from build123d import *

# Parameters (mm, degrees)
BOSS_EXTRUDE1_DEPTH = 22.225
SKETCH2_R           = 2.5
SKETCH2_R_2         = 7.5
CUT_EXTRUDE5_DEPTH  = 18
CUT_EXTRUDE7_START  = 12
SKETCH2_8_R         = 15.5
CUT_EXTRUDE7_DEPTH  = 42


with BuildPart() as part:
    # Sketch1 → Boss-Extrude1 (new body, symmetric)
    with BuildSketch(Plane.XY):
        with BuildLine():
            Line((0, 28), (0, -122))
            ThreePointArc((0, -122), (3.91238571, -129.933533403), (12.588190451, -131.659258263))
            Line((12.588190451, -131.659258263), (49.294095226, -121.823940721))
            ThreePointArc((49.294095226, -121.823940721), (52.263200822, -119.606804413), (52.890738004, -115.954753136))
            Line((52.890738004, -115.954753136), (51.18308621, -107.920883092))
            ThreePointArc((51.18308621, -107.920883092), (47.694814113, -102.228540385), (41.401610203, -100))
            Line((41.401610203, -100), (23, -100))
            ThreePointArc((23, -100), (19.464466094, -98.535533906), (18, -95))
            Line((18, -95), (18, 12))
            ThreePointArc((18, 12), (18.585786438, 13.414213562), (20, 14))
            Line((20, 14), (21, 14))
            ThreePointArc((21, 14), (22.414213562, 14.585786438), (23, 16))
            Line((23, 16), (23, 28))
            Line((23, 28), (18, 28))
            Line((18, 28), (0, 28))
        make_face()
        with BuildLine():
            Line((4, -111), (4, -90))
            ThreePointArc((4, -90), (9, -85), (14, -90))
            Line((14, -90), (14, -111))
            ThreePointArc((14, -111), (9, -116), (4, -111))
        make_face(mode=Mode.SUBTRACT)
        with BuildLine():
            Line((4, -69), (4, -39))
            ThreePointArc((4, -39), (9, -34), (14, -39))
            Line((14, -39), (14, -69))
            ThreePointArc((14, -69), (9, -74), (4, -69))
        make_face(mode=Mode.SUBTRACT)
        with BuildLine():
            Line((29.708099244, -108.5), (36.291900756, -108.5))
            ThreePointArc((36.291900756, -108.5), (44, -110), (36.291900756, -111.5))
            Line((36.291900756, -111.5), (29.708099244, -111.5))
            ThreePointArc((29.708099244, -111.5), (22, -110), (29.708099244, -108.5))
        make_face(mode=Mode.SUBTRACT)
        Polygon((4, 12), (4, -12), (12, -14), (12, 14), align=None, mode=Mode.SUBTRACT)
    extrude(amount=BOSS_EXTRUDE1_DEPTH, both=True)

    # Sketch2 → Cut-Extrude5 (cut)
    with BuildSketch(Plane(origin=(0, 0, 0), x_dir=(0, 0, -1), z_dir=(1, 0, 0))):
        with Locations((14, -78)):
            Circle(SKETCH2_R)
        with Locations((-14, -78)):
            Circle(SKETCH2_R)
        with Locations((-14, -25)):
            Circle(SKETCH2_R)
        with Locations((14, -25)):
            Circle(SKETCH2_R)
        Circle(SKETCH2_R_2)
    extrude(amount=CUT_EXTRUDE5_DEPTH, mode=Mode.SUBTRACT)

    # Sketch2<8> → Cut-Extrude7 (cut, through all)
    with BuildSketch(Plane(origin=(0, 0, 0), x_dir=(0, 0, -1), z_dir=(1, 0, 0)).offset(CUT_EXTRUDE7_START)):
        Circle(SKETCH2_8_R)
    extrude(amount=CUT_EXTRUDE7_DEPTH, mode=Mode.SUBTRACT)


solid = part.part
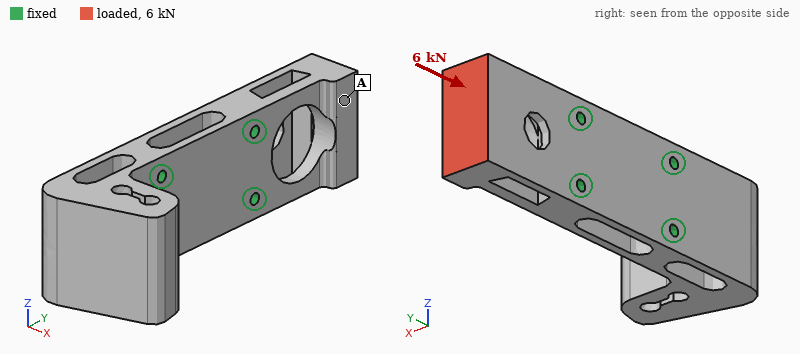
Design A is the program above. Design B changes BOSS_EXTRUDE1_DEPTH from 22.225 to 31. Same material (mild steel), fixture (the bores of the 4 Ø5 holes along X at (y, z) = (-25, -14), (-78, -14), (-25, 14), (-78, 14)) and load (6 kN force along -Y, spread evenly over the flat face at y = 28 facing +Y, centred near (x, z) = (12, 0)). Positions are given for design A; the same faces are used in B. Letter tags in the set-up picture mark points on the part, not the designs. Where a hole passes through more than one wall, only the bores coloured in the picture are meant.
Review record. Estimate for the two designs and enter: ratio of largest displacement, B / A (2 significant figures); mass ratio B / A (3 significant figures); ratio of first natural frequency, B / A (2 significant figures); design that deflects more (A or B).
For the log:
0.54
1.42
0.98
A
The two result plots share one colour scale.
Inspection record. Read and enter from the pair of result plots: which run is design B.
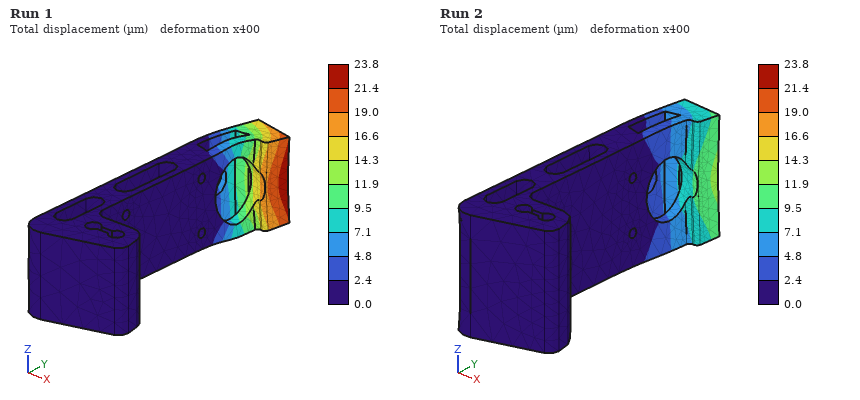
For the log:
Run 2
